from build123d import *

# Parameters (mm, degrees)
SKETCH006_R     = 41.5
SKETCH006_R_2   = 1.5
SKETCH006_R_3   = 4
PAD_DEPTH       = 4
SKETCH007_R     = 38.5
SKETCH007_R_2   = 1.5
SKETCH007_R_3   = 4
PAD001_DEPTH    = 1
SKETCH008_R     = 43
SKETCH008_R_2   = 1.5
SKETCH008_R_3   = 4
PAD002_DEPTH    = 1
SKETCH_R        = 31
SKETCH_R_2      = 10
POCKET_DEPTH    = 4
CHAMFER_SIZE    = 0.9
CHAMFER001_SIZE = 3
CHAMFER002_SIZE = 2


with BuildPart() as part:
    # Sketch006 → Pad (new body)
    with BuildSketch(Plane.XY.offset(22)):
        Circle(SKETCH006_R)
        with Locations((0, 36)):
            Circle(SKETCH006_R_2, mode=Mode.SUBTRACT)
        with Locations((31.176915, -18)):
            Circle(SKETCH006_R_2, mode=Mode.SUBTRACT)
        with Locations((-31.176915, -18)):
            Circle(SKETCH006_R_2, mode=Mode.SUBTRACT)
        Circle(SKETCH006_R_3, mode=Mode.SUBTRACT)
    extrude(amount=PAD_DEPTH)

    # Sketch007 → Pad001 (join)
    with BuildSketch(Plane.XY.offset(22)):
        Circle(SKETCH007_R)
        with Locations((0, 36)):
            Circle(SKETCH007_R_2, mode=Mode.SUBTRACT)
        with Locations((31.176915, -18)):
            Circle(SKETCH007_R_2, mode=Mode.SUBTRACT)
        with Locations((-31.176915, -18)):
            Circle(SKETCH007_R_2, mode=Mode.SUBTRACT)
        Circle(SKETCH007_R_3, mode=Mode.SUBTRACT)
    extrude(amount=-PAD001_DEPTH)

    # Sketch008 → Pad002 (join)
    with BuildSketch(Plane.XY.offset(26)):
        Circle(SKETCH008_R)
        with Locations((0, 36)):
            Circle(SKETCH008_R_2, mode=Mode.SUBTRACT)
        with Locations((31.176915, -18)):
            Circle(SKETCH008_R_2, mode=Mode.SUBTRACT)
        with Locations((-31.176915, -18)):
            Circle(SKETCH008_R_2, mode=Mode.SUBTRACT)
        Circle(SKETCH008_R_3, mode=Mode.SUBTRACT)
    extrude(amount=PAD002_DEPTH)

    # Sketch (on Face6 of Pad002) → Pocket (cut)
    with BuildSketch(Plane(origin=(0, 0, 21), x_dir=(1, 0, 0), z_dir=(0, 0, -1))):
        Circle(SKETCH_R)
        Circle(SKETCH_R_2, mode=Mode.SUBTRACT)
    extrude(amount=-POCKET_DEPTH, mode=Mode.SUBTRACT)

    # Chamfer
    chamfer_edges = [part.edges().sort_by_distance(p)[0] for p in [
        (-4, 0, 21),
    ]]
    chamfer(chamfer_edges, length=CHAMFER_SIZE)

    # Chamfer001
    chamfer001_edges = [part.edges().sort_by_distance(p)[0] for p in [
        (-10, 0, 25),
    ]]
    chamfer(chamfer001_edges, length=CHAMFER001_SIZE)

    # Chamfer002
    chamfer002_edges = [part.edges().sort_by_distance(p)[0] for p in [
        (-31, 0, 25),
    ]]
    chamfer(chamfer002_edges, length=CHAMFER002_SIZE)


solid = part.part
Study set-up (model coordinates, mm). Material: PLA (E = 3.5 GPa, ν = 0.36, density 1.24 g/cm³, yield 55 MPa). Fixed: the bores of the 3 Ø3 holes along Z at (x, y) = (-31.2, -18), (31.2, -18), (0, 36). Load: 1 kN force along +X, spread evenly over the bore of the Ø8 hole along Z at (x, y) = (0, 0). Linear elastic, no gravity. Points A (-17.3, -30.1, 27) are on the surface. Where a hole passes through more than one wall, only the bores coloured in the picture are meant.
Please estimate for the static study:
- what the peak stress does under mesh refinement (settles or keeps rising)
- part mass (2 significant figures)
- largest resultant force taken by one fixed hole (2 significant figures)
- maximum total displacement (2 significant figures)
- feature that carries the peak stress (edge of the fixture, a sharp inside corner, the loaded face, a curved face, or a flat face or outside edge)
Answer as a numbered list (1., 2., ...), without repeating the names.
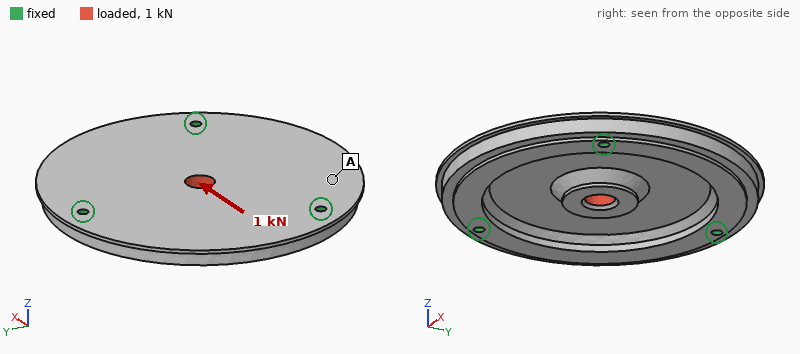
1. keeps rising
2. 27 g
3. 340 N
4. 0.20 mm
5. edge of the fixture
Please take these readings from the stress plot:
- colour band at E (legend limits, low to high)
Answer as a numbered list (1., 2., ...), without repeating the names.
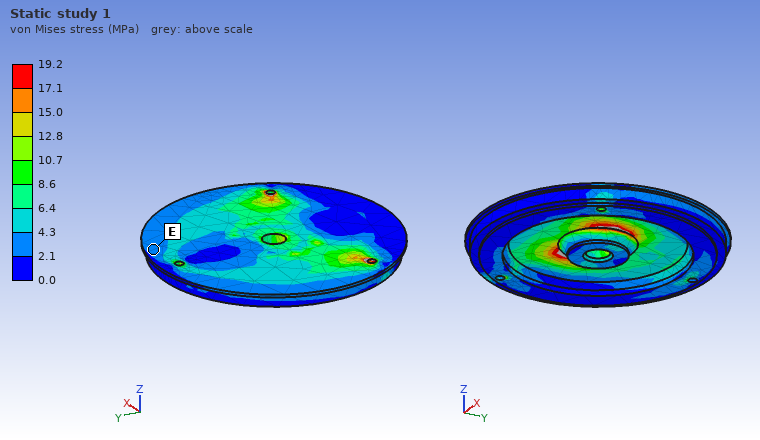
1. 2.1 to 4.3 MPa
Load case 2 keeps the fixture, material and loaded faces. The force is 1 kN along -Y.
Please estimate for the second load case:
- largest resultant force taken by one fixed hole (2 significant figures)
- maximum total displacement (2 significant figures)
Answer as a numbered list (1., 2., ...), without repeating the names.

1. 340 N
2. 0.20 mm
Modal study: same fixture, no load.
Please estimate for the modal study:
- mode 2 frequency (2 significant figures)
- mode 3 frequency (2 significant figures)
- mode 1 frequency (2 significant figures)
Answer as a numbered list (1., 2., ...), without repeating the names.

1. 1500 Hz
2. 1500 Hz
3. 1500 Hz
